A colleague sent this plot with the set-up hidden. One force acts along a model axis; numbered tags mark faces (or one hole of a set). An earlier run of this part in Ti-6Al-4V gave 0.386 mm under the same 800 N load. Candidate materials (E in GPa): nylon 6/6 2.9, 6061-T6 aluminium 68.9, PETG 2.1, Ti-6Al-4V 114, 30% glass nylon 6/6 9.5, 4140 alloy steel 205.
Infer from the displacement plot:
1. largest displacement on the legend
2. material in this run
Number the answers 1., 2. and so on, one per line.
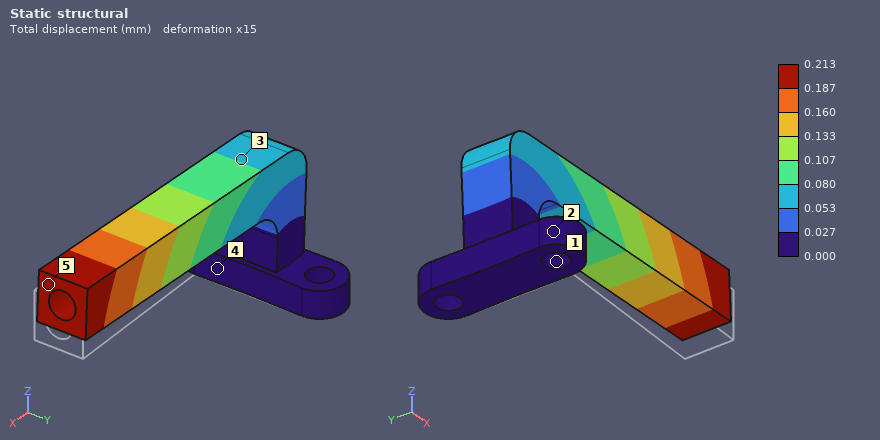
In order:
1. 0.213 mm
2. 4140 alloy steel
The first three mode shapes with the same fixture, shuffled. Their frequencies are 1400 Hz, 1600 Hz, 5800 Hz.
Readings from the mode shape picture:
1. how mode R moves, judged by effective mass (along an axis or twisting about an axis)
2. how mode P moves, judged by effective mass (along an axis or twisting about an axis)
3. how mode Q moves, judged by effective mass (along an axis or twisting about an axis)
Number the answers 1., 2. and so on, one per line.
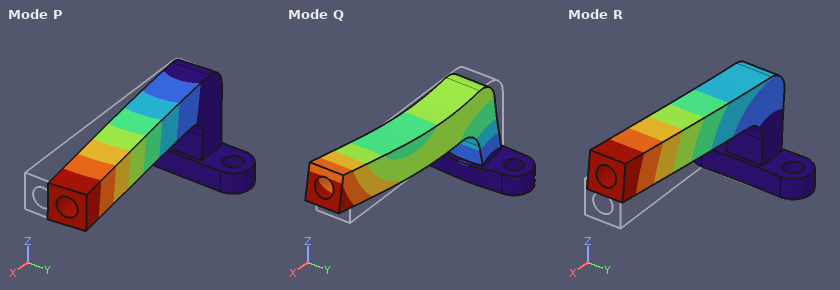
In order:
1. along Z
2. along Y
3. along X
